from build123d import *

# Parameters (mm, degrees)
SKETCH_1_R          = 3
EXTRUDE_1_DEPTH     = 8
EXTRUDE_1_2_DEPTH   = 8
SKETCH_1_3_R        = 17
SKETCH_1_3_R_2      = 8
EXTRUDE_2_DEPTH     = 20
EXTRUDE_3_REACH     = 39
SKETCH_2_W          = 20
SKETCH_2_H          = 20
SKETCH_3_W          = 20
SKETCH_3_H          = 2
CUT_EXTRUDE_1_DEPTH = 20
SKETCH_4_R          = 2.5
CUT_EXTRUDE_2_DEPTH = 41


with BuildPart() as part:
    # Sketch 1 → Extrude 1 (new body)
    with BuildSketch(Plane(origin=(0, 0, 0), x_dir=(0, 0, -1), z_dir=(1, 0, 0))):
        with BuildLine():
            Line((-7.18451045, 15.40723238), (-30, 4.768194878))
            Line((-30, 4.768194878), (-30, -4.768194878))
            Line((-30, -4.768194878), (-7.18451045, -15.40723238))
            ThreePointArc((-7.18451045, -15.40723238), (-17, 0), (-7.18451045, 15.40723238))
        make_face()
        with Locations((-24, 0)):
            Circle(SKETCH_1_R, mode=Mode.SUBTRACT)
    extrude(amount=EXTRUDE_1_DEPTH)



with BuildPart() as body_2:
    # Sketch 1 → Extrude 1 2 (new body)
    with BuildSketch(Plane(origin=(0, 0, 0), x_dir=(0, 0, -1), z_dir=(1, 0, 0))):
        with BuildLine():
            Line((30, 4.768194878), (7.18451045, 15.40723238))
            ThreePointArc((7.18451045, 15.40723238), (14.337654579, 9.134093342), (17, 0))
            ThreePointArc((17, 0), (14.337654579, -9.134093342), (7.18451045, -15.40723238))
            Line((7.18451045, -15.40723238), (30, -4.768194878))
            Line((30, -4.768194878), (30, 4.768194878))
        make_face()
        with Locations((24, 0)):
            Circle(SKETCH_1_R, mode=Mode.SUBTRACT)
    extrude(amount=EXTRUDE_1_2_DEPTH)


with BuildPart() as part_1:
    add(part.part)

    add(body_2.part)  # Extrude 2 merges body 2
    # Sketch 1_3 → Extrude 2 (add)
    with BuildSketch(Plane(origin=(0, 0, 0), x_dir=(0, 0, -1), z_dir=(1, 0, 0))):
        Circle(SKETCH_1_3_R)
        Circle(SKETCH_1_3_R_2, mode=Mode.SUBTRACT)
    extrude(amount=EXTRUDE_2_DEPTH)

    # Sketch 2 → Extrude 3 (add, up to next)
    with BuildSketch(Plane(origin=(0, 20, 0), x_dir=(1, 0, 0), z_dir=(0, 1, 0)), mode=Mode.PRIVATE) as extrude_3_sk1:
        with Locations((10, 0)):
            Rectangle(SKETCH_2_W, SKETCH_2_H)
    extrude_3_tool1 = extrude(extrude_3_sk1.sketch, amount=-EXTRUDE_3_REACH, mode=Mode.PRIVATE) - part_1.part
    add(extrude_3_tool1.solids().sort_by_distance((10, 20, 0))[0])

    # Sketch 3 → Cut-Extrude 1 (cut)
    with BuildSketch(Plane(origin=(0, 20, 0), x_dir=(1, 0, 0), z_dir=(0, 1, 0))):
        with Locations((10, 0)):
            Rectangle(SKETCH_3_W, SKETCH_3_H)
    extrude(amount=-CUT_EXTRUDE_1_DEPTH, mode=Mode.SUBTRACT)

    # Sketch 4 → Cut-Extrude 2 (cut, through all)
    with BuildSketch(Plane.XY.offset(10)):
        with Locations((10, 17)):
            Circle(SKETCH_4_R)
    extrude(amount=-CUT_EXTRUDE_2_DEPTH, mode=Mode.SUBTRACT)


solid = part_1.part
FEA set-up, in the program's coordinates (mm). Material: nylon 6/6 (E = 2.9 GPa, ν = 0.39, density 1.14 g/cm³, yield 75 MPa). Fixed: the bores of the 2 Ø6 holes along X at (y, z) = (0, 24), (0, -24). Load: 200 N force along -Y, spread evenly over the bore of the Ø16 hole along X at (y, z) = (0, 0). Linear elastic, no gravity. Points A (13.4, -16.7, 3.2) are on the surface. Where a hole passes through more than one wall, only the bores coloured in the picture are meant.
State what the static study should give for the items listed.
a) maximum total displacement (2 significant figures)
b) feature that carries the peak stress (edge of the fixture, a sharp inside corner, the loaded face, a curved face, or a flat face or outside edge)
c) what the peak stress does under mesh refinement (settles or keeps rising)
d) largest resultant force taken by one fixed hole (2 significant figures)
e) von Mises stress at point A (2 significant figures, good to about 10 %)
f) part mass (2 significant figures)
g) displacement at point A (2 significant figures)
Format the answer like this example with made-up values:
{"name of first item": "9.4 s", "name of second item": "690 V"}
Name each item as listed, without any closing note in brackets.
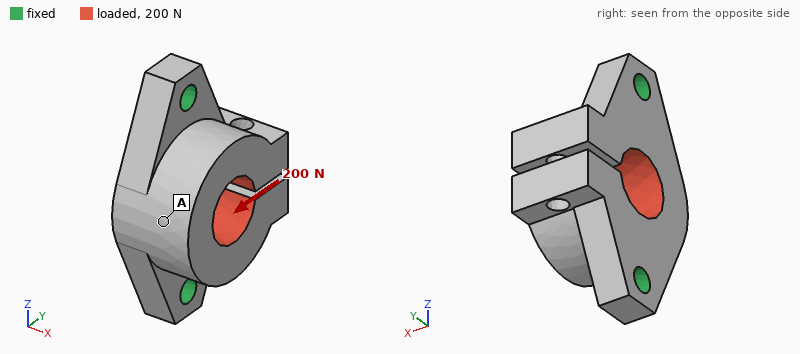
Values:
{"maximum total displacement": "73 µm", "feature that carries the peak stress": "edge of the fixture", "what the peak stress does under mesh refinement": "keeps rising", "largest resultant force taken by one fixed hole": "130 N", "von Mises stress at point A": "0.54 MPa", "part mass": "21 g", "displacement at point A": "51 µm"}
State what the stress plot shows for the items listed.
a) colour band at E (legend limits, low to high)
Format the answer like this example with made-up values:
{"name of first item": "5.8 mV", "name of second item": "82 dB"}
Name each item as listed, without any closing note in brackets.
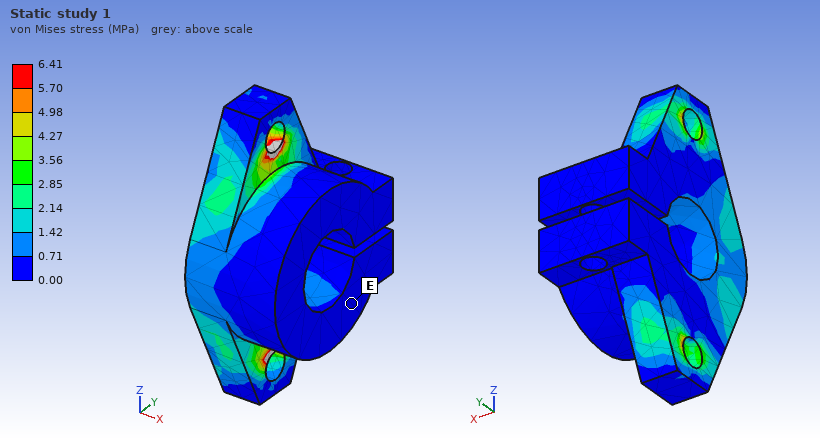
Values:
{"colour band at E": "0.00 to 0.71 MPa"}
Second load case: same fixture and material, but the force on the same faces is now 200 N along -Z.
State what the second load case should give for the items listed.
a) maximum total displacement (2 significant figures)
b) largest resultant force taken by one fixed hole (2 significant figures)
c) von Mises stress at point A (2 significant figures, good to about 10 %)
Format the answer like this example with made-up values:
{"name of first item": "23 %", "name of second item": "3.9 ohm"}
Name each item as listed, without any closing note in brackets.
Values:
{"maximum total displacement": "29 µm", "largest resultant force taken by one fixed hole": "100 N", "von Mises stress at point A": "0.32 MPa"}
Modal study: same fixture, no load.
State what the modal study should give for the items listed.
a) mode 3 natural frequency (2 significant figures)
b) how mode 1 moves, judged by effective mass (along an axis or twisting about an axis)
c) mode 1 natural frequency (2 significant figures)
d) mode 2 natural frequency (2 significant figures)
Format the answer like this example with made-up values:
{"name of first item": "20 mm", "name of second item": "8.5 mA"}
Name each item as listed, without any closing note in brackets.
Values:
{"mode 3 natural frequency": "2800 Hz", "how mode 1 moves, judged by effective mass": "along Y", "mode 1 natural frequency": "2200 Hz", "mode 2 natural frequency": "2600 Hz"}
